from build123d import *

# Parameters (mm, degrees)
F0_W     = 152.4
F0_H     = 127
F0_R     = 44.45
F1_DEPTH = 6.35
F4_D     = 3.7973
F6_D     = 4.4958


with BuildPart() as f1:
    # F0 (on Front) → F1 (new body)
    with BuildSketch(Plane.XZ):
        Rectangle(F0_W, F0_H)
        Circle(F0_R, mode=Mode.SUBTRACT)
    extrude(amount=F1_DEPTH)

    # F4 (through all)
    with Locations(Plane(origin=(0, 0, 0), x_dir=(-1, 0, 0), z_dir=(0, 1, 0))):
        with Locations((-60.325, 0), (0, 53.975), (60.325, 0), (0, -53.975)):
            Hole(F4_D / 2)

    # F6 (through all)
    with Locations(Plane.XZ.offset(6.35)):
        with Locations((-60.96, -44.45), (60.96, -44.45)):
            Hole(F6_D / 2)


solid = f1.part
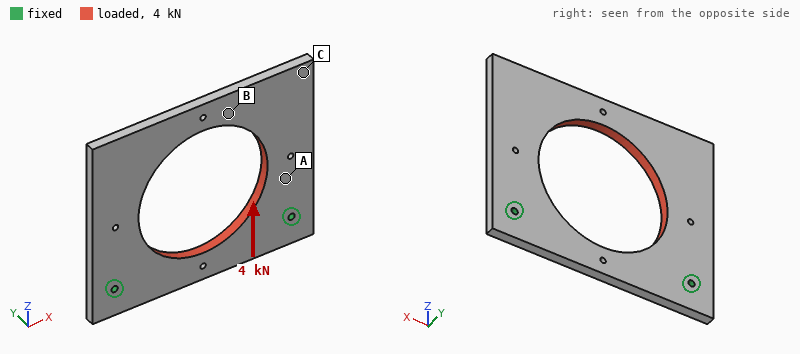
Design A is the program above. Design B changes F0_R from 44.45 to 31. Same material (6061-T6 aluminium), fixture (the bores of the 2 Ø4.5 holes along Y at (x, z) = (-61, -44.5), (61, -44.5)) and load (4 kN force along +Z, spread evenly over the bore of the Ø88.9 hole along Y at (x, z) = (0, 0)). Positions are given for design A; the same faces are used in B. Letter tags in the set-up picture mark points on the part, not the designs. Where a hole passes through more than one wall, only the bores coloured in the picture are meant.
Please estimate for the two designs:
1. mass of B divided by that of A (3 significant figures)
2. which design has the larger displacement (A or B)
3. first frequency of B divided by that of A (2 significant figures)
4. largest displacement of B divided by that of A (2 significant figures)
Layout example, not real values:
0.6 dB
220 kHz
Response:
1.24
A
1.0
0.76
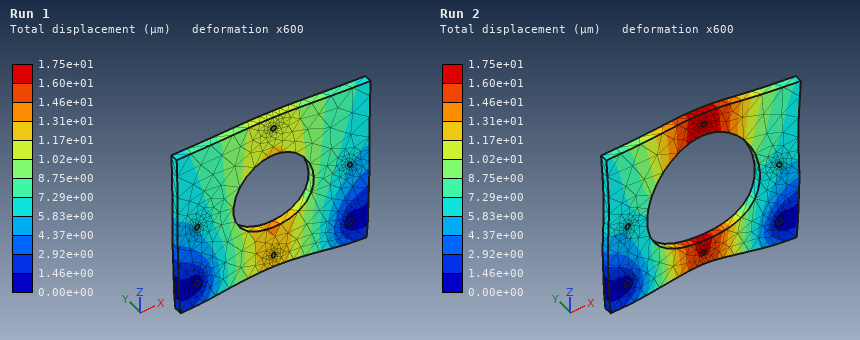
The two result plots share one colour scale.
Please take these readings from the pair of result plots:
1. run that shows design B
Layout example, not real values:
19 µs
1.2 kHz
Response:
Run 1
